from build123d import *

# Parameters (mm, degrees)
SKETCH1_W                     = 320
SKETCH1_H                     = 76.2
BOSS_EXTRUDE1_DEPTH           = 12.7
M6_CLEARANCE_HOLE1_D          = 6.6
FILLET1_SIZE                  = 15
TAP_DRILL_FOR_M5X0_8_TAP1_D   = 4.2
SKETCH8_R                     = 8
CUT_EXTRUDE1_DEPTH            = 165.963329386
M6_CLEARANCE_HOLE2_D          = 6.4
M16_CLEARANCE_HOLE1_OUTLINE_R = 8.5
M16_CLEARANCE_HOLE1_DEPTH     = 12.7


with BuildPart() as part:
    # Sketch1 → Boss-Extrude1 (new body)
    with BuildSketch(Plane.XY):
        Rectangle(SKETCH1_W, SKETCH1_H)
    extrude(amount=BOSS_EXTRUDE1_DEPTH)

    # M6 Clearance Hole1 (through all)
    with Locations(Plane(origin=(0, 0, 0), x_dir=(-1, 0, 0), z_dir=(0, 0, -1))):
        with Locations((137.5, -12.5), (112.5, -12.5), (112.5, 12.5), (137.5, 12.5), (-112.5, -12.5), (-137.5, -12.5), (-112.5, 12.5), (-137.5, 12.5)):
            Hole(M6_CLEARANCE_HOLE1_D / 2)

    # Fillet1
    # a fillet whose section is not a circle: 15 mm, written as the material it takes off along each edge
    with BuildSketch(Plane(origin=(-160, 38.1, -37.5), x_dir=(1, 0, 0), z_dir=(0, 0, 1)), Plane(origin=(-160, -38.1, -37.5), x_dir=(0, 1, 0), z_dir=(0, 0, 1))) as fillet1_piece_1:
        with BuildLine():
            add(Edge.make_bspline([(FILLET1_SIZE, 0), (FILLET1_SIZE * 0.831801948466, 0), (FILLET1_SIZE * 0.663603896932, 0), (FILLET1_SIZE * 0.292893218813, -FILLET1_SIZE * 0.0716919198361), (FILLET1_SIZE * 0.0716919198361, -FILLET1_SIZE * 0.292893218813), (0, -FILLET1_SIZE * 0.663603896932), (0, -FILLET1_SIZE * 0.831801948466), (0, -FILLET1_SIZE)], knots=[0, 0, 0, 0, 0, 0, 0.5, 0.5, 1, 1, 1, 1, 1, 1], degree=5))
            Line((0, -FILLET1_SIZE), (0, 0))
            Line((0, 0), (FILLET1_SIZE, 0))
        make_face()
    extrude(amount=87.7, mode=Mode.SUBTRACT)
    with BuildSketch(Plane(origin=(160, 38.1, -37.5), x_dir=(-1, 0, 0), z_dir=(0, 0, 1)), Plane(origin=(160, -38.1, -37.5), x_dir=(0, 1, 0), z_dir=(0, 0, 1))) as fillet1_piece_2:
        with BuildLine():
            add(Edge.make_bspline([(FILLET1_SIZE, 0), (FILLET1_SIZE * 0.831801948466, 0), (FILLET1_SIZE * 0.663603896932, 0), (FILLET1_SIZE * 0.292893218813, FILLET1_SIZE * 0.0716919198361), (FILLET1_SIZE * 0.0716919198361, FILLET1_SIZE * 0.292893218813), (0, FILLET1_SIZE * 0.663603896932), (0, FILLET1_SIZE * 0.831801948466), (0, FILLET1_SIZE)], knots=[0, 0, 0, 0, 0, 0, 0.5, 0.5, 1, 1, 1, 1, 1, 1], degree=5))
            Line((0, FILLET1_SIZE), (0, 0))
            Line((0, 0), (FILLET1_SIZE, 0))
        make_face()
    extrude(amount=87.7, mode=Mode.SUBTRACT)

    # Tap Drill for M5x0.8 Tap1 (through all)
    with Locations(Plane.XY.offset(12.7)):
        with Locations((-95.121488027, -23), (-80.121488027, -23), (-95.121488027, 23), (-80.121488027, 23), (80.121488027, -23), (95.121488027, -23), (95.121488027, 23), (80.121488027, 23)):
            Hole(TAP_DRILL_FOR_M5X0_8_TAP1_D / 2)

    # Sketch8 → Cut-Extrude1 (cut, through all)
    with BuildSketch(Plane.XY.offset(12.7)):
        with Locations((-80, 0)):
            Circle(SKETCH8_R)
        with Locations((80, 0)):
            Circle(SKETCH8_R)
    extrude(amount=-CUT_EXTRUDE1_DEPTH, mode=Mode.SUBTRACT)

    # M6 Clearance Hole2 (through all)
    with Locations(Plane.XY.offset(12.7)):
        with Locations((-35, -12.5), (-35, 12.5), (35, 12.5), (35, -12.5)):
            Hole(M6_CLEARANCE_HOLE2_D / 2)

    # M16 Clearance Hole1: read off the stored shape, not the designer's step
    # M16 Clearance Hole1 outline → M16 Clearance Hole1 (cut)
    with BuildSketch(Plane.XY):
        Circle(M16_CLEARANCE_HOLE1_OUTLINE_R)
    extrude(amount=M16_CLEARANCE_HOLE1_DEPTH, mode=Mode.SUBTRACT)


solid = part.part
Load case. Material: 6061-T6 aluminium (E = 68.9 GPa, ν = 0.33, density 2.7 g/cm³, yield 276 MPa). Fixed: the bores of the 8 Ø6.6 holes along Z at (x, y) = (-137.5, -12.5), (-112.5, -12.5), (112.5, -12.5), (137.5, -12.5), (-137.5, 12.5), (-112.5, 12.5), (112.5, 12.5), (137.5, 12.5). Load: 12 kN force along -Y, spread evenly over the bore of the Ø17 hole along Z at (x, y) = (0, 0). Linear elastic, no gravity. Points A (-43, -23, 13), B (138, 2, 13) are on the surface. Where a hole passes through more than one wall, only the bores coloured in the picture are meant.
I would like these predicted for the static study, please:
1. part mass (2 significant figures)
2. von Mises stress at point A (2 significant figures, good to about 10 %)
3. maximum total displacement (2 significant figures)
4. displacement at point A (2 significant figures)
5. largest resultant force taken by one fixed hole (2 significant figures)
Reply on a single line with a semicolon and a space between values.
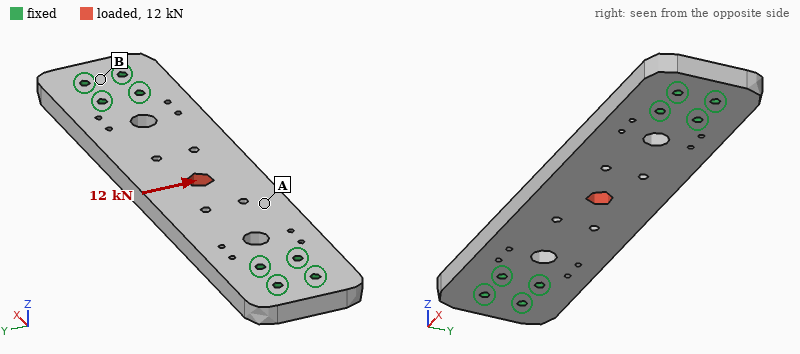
790 g; 11 MPa; 73 µm; 52 µm; 6.2 kN
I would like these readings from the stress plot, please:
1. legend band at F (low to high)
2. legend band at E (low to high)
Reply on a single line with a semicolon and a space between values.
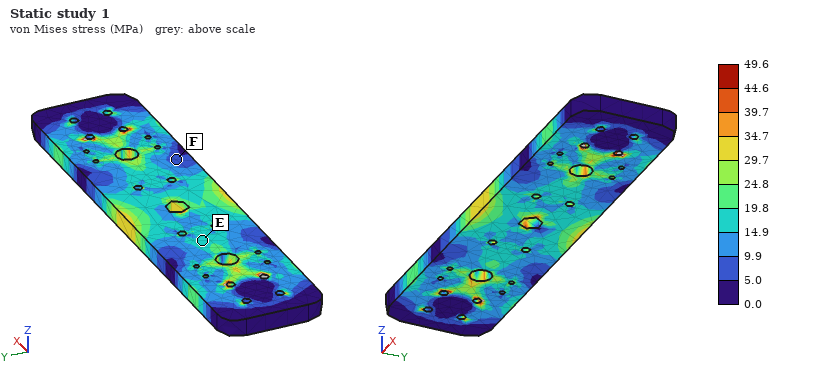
5.0 to 9.9 MPa; 14.9 to 19.8 MPa
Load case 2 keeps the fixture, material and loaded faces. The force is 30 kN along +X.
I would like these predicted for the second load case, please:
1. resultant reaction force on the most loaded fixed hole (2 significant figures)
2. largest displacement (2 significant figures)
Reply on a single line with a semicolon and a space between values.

5.8 kN; 39 µm
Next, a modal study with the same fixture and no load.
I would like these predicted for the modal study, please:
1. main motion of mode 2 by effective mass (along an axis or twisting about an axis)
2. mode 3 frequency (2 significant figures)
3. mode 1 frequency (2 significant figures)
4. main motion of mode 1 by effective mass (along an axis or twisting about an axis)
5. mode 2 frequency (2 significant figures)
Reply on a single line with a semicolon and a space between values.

twisting about X; 3300 Hz; 1200 Hz; along Z; 2300 Hz
